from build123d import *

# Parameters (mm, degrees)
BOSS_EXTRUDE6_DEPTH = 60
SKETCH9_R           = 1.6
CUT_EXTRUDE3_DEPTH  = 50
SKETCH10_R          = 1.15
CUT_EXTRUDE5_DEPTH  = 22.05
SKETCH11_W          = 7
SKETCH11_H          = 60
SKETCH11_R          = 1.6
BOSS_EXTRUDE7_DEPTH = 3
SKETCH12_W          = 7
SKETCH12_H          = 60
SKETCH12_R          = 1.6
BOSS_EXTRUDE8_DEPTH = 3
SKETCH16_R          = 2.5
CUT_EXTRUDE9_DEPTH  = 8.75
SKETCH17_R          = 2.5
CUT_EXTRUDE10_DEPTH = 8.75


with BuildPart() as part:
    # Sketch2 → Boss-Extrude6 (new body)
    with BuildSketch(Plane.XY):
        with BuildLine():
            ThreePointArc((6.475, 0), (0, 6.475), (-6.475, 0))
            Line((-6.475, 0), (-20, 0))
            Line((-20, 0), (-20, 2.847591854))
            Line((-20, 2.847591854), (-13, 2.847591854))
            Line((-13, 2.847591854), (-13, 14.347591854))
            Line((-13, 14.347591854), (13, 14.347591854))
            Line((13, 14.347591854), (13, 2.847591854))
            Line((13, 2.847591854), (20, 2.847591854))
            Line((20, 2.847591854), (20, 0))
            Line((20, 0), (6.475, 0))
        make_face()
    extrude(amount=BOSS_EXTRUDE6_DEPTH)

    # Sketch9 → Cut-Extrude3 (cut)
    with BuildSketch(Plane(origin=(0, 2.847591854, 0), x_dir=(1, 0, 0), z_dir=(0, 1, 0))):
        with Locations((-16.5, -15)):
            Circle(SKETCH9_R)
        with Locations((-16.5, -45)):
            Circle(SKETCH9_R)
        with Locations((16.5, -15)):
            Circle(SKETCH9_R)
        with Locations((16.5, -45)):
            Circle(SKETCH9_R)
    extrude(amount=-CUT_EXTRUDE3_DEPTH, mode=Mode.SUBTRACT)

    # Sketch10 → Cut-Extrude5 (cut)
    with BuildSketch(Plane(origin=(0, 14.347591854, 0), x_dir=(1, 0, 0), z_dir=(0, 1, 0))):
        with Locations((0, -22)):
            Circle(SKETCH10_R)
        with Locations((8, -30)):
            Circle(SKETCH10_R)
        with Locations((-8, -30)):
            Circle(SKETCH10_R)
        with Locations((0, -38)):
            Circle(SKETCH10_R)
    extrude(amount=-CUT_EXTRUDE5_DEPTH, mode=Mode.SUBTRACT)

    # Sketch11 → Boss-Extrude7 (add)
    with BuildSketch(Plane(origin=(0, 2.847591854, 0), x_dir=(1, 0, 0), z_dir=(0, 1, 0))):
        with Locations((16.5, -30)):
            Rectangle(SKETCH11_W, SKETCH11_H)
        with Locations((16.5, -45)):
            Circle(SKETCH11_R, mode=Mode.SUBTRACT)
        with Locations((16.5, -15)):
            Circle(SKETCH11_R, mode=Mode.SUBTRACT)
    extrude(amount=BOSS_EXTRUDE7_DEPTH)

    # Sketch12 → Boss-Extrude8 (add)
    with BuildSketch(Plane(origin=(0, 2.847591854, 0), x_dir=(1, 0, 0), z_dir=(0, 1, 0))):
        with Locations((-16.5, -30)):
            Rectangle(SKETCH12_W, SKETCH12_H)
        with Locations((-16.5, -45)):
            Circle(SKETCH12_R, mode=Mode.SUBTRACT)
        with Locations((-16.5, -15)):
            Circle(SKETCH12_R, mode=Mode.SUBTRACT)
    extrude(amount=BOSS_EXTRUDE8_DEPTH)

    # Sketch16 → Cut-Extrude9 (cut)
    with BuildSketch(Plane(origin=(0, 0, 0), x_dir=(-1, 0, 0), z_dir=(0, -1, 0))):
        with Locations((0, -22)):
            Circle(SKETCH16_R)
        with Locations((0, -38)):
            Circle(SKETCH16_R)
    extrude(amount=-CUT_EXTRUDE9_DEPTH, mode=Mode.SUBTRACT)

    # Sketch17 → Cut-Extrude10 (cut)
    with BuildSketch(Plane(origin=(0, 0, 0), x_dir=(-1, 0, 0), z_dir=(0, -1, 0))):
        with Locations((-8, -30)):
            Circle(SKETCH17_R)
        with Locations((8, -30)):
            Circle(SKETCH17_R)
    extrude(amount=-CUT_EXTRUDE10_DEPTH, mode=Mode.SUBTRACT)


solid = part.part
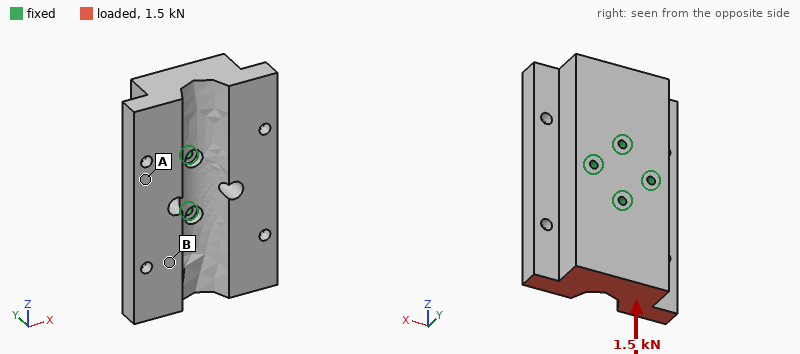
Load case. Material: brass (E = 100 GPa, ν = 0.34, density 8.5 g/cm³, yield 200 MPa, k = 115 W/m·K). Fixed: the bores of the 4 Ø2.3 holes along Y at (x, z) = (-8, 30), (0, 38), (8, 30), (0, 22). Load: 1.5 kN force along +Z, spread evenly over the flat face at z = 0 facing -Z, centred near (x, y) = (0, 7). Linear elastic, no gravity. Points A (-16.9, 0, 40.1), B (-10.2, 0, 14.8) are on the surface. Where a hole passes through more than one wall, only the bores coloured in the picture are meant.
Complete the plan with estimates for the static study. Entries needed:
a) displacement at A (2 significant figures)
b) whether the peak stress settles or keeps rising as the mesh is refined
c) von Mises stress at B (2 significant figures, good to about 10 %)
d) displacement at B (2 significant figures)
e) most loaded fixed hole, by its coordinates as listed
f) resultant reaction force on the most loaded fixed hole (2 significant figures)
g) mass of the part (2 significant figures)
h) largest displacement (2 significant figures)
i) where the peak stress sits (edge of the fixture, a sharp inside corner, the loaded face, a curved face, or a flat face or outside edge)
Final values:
1.7 µm
keeps rising
4.2 MPa
2.7 µm
(0, 22)
580 N
190 g
4.6 µm
edge of the fixture
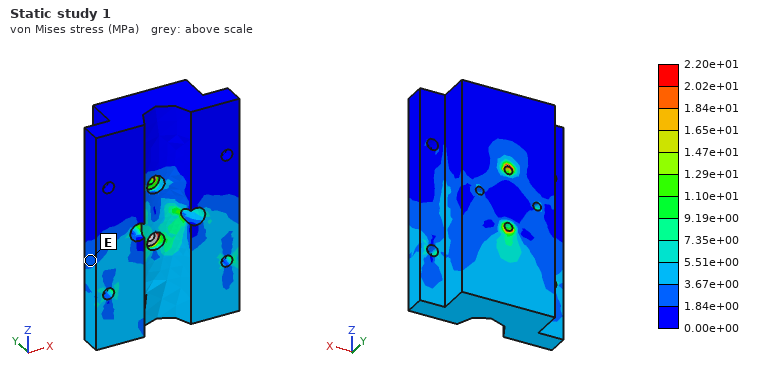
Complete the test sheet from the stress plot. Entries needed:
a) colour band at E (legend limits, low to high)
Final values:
1.84e+00 to 3.67e+00 MPa
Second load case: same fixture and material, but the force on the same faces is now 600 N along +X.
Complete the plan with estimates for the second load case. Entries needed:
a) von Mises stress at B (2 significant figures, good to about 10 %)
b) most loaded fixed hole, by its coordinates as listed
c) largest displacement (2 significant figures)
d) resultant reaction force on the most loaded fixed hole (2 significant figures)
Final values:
3.7 MPa
(0, 22)
7.9 µm
740 N
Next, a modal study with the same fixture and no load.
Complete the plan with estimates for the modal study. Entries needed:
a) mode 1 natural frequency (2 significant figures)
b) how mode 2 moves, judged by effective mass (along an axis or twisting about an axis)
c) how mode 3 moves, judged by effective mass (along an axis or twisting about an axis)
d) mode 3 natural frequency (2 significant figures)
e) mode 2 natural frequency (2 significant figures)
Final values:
5100 Hz
along X
twisting about Y
7100 Hz
6700 Hz
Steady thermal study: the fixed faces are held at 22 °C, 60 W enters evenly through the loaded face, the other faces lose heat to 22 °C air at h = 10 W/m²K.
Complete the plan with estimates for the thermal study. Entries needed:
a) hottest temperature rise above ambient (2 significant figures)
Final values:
42 K
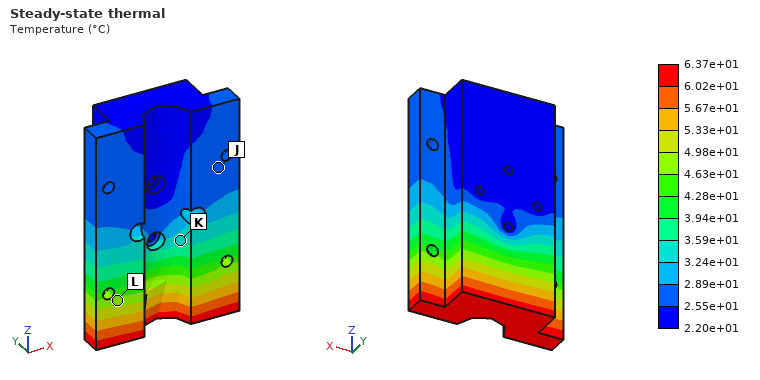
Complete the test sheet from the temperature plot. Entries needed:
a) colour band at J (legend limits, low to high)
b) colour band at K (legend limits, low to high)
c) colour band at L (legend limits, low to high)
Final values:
2.55e+01 to 2.89e+01 °C
3.24e+01 to 3.59e+01 °C
4.63e+01 to 4.98e+01 °C
